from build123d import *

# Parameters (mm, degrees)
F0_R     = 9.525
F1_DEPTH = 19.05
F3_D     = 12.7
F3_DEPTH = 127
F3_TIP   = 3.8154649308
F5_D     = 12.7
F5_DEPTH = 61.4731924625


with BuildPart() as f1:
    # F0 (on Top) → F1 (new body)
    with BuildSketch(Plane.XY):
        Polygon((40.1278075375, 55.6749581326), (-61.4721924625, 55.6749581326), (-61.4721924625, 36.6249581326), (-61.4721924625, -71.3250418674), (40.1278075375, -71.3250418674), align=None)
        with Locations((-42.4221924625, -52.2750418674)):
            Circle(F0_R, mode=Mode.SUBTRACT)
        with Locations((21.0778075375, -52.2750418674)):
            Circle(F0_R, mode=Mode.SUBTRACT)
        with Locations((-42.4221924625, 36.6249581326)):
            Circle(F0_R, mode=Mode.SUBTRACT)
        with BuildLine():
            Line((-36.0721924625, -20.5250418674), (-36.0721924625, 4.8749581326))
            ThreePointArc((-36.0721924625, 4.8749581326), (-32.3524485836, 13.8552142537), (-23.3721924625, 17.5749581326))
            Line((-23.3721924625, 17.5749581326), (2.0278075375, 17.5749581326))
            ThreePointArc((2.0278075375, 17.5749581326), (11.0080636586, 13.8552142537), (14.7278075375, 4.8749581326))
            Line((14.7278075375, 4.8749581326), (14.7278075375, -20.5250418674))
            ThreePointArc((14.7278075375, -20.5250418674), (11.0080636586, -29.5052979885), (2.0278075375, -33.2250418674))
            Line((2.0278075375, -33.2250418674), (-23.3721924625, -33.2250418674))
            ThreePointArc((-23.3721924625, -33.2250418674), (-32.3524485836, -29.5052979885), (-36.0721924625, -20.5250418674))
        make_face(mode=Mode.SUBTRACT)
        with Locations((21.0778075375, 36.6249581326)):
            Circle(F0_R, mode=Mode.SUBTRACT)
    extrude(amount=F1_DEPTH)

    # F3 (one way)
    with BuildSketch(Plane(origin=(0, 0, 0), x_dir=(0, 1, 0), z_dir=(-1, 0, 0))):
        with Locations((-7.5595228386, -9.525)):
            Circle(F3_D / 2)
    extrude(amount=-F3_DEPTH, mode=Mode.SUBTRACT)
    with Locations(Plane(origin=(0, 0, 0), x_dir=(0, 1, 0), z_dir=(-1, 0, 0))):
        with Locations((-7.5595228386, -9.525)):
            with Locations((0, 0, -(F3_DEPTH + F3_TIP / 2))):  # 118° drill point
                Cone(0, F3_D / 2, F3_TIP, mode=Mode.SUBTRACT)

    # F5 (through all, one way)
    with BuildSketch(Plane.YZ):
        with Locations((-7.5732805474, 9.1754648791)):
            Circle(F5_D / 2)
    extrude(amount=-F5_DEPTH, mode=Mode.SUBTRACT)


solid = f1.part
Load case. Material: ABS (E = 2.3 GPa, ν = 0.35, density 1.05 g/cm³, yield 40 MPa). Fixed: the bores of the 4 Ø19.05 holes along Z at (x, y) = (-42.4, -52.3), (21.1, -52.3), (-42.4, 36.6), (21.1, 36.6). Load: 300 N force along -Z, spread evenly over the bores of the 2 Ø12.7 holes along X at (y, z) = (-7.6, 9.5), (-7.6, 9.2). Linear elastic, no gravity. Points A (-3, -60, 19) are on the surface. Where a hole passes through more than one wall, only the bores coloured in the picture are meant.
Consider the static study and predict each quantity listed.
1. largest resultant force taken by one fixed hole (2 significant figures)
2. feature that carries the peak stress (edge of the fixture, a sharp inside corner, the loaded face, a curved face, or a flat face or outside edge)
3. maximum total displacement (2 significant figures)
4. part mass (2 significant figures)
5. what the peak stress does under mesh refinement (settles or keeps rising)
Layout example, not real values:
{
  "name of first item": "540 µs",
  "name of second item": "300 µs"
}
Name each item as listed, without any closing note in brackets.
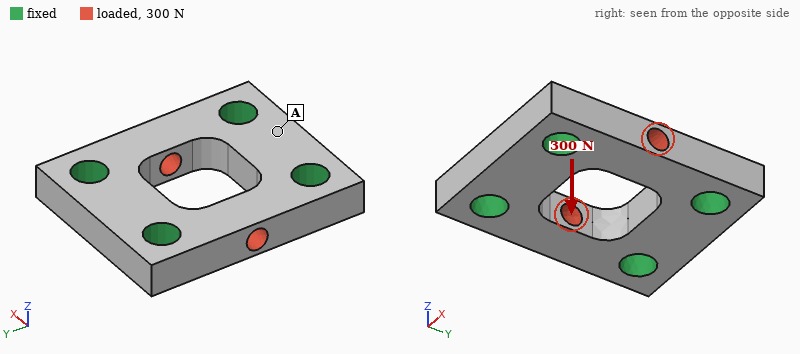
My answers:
{
  "largest resultant force taken by one fixed hole": "76 N",
  "feature that carries the peak stress": "edge of the fixture",
  "maximum total displacement": "18 µm",
  "part mass": "180 g",
  "what the peak stress does under mesh refinement": "keeps rising"
}
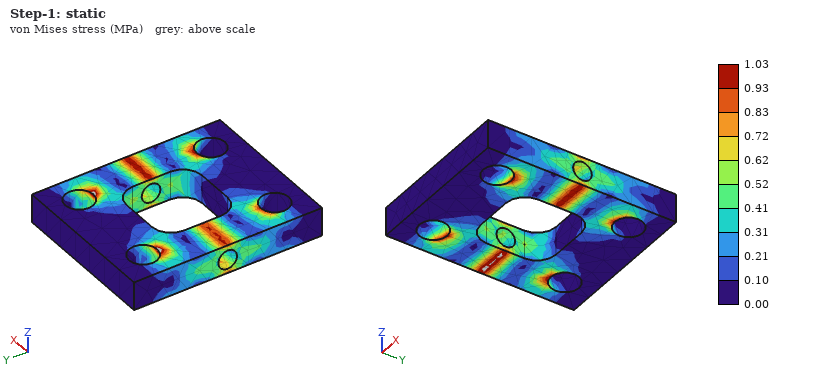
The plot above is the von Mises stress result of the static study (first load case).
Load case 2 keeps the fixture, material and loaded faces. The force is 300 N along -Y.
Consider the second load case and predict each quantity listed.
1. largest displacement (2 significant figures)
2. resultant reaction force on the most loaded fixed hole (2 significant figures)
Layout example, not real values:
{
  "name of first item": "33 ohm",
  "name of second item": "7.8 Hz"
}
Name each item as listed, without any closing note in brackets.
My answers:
{
  "largest displacement": "2.6 µm",
  "resultant reaction force on the most loaded fixed hole": "75 N"
}
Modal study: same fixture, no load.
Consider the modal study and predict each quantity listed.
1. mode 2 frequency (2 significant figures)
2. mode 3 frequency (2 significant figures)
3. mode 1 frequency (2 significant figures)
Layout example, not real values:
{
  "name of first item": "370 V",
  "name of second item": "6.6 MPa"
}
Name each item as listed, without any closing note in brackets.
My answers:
{
  "mode 2 frequency": "4300 Hz",
  "mode 3 frequency": "5100 Hz",
  "mode 1 frequency": "4300 Hz"
}
